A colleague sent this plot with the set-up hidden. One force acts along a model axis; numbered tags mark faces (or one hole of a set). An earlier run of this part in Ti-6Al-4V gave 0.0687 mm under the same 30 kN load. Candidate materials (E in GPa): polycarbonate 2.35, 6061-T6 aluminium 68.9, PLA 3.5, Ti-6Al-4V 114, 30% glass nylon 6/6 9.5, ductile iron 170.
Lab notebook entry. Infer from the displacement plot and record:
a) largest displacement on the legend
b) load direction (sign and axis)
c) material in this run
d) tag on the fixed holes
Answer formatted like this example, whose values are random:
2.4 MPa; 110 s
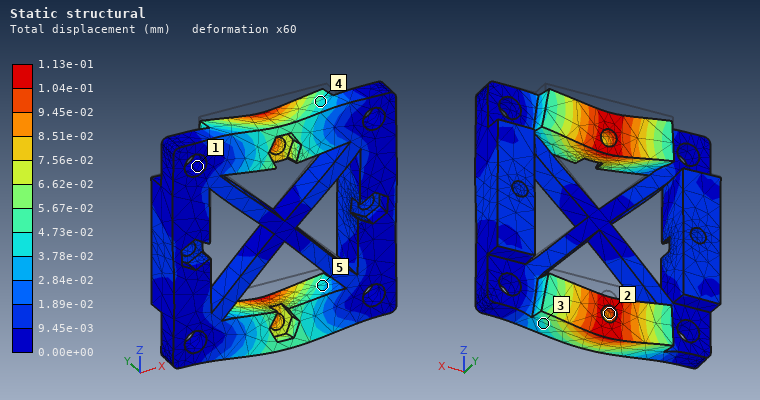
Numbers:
1.13e-01 mm; -Z; 6061-T6 aluminium; 1
